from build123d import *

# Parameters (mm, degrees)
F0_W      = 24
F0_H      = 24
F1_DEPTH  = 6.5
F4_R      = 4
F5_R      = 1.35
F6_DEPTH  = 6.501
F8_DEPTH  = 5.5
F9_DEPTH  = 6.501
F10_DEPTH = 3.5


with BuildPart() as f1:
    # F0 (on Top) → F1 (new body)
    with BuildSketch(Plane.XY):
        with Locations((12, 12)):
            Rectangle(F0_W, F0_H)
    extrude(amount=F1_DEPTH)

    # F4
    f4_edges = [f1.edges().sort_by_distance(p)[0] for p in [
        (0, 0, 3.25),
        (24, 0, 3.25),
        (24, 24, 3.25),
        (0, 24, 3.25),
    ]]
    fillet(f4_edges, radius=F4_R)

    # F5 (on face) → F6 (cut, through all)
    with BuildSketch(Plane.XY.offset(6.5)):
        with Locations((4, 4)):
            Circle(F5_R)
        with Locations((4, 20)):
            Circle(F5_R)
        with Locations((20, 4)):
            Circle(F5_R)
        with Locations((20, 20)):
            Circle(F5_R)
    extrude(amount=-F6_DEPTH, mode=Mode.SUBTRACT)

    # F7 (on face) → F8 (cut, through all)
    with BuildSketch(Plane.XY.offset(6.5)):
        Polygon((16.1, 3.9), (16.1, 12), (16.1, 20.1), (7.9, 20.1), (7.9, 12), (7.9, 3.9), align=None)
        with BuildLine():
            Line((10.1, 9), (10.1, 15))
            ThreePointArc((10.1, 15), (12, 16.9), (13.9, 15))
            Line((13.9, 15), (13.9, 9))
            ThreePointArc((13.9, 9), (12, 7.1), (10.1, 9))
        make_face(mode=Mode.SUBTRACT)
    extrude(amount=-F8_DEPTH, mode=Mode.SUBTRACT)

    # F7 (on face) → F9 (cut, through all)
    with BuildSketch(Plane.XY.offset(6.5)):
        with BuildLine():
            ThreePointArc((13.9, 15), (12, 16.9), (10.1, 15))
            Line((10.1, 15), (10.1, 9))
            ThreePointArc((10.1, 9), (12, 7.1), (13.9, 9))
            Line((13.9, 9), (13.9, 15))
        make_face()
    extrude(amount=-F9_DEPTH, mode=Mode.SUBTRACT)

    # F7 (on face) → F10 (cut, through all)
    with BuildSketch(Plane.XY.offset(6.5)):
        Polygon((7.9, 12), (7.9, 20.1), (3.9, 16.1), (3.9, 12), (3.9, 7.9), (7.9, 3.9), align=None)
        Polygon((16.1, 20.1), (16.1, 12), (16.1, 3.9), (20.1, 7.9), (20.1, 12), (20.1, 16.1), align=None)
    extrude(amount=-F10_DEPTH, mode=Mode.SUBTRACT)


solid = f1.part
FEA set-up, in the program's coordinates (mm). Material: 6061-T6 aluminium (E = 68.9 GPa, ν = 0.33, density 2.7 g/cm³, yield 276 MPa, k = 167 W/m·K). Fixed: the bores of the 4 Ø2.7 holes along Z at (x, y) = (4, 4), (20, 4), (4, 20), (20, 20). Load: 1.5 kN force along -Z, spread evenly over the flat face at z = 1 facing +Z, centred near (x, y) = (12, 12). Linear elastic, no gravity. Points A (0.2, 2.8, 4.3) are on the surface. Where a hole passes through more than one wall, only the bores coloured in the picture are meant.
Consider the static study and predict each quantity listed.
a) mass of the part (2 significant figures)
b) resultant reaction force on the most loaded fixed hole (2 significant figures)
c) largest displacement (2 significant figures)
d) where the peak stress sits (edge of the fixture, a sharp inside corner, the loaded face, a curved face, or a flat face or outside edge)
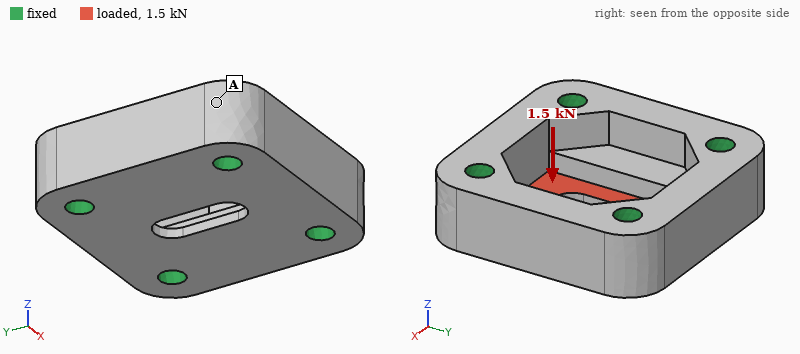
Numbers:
6.5 g
390 N
37 µm
a curved face
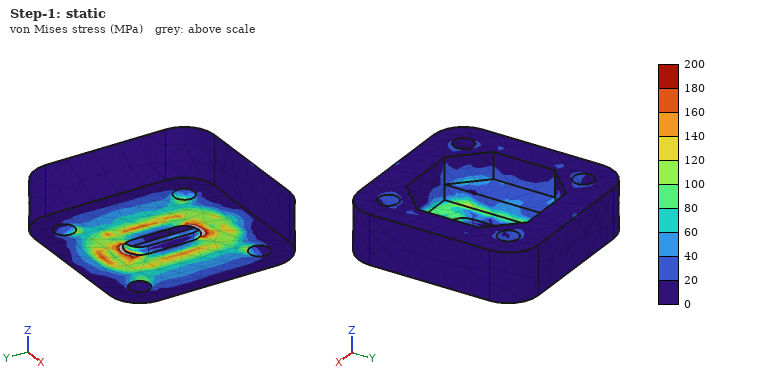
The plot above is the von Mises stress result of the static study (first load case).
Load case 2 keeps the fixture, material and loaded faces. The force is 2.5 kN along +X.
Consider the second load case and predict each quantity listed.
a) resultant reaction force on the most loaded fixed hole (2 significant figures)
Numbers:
640 N
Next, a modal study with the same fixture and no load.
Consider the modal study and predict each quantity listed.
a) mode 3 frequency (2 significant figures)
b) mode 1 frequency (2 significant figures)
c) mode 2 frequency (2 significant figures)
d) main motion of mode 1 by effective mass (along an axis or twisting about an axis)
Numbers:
76 kHz
63 kHz
66 kHz
along Z
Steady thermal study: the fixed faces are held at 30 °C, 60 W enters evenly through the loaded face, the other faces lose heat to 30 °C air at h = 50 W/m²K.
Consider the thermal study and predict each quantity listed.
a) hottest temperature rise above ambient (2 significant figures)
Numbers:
29 K
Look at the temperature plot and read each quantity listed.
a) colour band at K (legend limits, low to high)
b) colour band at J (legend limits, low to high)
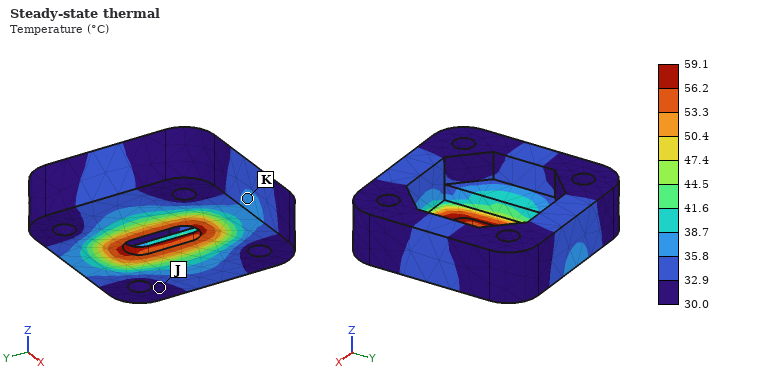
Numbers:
35.8 to 38.7 °C
30.0 to 32.9 °C
